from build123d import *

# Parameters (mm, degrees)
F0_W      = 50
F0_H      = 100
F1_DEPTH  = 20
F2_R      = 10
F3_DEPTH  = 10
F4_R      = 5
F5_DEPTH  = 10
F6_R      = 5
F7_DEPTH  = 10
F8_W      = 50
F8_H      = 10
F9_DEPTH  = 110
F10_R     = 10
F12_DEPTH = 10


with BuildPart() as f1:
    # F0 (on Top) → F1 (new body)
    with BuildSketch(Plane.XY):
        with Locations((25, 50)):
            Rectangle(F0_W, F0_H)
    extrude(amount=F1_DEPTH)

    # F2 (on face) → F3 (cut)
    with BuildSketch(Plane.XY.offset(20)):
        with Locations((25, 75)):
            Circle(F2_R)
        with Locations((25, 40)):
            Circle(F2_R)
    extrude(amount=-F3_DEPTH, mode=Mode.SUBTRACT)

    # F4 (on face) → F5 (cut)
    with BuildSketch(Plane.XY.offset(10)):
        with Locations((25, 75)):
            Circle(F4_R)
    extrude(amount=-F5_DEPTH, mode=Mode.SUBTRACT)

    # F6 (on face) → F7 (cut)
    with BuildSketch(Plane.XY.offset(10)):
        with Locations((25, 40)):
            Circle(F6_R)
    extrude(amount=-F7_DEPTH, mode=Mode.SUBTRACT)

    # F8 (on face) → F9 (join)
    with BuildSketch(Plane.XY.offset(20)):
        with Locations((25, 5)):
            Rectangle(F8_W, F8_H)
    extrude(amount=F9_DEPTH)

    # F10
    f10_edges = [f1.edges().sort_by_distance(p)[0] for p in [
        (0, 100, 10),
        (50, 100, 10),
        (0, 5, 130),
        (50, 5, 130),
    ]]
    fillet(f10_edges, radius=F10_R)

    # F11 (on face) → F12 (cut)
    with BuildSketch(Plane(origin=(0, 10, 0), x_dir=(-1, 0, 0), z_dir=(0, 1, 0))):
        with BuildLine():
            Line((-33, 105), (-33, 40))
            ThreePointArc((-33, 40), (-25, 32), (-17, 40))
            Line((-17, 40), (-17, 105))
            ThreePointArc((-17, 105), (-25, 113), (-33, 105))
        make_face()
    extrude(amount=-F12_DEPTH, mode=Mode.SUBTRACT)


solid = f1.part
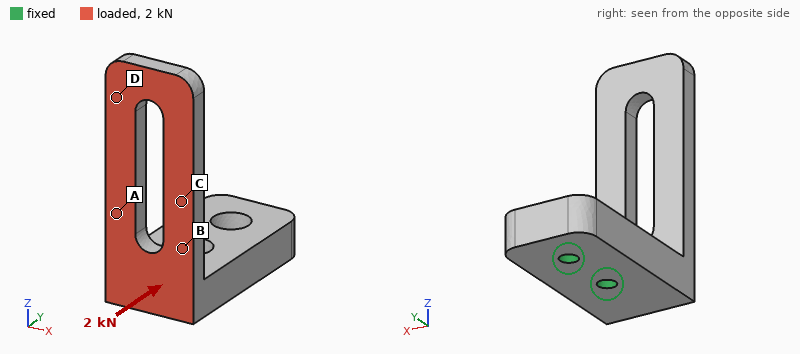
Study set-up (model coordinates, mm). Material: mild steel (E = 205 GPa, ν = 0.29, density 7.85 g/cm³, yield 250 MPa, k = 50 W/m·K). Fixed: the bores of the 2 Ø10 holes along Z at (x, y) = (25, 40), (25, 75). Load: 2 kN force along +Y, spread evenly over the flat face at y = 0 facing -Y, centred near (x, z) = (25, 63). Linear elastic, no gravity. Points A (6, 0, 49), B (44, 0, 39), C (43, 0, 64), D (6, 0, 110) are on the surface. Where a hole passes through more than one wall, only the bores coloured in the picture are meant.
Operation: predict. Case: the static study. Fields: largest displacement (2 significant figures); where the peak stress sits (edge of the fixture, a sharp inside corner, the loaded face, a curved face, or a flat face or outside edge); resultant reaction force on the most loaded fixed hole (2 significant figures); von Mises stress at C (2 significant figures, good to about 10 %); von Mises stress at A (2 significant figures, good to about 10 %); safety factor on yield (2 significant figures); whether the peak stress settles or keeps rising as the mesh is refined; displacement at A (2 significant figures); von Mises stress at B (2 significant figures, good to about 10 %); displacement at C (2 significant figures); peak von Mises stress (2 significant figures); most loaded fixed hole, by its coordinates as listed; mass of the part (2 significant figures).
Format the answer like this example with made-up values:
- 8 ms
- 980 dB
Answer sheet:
- 0.58 mm
- a curved face
- 3.5 kN
- 61 MPa
- 88 MPa
- 1.7
- settles
- 0.097 mm
- 100 MPa
- 0.17 mm
- 150 MPa
- (25, 75)
- 1.0 kg
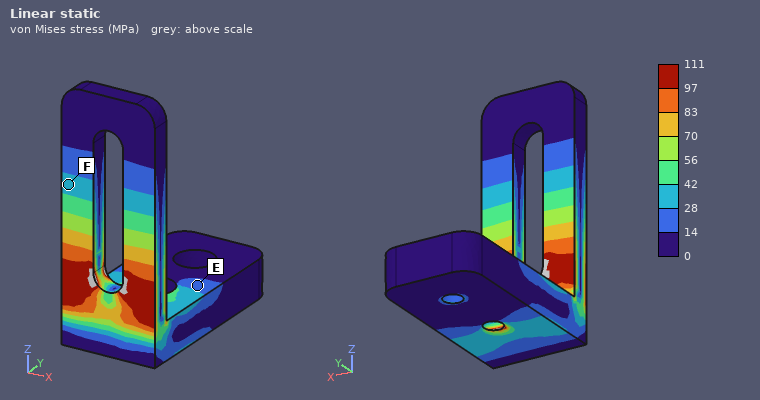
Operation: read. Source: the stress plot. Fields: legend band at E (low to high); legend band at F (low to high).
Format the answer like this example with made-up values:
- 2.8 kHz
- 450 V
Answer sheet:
- 14 to 28 MPa
- 28 to 42 MPa
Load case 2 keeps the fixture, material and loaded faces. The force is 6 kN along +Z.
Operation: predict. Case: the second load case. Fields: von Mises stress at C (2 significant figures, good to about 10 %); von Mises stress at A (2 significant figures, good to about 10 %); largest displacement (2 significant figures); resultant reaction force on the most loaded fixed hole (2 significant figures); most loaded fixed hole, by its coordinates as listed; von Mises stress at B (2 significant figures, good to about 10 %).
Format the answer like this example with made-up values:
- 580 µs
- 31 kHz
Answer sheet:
- 34 MPa
- 40 MPa
- 0.32 mm
- 11 kN
- (25, 40)
- 43 MPa
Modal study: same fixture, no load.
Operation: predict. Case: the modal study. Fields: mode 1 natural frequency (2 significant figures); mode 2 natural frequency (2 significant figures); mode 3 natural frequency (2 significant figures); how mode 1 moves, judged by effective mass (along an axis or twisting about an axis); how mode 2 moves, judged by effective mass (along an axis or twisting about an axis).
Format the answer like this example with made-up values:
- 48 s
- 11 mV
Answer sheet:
- 560 Hz
- 1000 Hz
- 2200 Hz
- along Y
- along X
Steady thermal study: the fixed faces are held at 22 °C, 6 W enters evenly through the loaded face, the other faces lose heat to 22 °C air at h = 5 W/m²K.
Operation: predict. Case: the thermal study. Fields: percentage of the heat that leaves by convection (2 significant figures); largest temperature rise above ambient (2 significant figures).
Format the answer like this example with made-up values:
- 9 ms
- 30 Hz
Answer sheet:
- 12 %
- 18 K
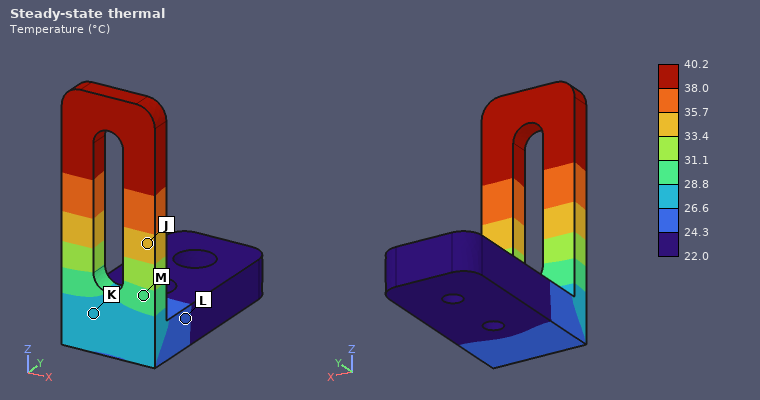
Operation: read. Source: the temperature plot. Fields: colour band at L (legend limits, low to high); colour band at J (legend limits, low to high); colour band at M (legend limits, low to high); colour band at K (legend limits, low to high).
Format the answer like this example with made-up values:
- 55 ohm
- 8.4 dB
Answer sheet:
- 24.3 to 26.6 °C
- 33.4 to 35.7 °C
- 28.8 to 31.1 °C
- 26.6 to 28.8 °C
